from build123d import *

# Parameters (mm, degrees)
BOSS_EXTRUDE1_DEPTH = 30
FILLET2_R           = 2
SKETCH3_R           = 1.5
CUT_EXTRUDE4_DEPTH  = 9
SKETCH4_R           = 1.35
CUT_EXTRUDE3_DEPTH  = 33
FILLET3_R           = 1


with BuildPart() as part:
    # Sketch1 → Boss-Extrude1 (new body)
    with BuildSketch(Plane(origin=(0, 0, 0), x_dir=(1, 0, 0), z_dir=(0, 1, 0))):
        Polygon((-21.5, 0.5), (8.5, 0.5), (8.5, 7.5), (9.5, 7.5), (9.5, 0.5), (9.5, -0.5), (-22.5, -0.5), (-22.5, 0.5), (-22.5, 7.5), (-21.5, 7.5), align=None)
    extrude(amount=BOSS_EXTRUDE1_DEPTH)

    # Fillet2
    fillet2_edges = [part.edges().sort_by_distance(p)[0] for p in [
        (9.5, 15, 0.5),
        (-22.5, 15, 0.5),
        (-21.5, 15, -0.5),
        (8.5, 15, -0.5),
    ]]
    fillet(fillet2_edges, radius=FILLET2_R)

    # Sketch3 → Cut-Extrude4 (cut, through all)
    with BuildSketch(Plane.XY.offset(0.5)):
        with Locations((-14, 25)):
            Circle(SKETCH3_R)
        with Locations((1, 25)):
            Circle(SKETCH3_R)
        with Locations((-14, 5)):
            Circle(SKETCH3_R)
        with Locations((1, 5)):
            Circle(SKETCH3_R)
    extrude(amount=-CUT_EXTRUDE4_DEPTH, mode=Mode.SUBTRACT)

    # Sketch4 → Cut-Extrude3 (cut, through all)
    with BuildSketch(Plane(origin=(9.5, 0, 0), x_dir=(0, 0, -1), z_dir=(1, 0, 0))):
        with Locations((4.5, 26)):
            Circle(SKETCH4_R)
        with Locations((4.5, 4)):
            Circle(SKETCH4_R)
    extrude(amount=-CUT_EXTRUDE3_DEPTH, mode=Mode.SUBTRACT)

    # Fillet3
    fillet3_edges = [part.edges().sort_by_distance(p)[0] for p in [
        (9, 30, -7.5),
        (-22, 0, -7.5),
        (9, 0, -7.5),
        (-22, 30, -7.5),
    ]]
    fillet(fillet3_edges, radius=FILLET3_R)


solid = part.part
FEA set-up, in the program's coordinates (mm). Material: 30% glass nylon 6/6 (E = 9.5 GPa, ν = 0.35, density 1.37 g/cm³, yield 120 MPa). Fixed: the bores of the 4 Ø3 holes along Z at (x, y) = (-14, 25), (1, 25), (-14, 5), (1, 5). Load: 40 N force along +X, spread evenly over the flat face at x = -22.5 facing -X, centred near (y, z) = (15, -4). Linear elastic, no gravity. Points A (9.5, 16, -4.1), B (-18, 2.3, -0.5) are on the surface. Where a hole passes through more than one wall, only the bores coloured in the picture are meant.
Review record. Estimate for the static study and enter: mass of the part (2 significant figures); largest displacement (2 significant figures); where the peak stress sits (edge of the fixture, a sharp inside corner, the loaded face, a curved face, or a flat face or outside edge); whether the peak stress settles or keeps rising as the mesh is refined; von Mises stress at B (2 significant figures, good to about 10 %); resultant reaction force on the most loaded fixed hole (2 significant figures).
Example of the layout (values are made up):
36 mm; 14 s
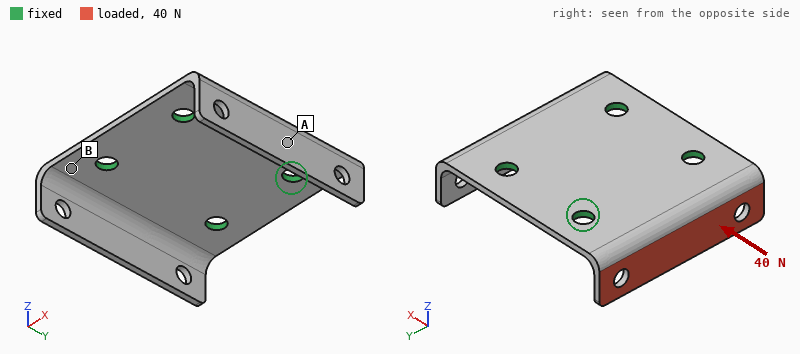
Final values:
1.8 g; 0.45 mm; edge of the fixture; keeps rising; 36 MPa; 16 N
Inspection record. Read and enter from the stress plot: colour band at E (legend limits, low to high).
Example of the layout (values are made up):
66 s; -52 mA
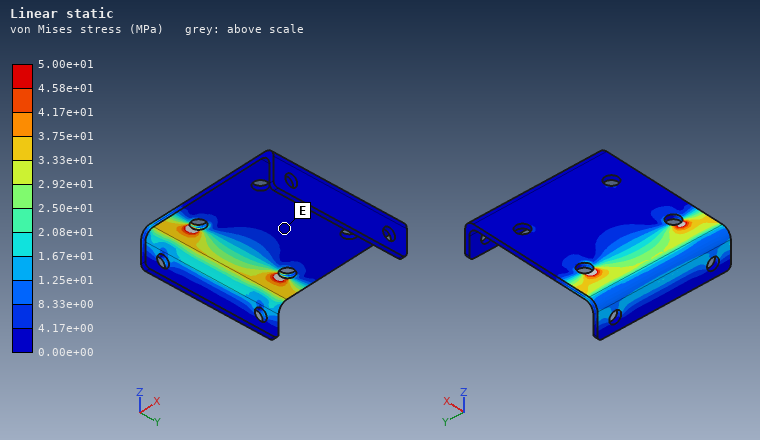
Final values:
0.00e+00 to 4.17e+00 MPa
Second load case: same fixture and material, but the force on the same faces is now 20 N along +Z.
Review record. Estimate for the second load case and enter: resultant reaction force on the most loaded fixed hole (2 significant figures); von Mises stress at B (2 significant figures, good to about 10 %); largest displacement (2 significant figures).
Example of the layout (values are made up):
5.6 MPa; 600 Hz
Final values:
11 N; 19 MPa; 0.24 mm
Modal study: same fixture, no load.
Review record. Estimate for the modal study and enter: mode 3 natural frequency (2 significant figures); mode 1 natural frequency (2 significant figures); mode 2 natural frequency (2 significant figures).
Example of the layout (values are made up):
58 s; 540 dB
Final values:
4100 Hz; 2700 Hz; 2800 Hz
